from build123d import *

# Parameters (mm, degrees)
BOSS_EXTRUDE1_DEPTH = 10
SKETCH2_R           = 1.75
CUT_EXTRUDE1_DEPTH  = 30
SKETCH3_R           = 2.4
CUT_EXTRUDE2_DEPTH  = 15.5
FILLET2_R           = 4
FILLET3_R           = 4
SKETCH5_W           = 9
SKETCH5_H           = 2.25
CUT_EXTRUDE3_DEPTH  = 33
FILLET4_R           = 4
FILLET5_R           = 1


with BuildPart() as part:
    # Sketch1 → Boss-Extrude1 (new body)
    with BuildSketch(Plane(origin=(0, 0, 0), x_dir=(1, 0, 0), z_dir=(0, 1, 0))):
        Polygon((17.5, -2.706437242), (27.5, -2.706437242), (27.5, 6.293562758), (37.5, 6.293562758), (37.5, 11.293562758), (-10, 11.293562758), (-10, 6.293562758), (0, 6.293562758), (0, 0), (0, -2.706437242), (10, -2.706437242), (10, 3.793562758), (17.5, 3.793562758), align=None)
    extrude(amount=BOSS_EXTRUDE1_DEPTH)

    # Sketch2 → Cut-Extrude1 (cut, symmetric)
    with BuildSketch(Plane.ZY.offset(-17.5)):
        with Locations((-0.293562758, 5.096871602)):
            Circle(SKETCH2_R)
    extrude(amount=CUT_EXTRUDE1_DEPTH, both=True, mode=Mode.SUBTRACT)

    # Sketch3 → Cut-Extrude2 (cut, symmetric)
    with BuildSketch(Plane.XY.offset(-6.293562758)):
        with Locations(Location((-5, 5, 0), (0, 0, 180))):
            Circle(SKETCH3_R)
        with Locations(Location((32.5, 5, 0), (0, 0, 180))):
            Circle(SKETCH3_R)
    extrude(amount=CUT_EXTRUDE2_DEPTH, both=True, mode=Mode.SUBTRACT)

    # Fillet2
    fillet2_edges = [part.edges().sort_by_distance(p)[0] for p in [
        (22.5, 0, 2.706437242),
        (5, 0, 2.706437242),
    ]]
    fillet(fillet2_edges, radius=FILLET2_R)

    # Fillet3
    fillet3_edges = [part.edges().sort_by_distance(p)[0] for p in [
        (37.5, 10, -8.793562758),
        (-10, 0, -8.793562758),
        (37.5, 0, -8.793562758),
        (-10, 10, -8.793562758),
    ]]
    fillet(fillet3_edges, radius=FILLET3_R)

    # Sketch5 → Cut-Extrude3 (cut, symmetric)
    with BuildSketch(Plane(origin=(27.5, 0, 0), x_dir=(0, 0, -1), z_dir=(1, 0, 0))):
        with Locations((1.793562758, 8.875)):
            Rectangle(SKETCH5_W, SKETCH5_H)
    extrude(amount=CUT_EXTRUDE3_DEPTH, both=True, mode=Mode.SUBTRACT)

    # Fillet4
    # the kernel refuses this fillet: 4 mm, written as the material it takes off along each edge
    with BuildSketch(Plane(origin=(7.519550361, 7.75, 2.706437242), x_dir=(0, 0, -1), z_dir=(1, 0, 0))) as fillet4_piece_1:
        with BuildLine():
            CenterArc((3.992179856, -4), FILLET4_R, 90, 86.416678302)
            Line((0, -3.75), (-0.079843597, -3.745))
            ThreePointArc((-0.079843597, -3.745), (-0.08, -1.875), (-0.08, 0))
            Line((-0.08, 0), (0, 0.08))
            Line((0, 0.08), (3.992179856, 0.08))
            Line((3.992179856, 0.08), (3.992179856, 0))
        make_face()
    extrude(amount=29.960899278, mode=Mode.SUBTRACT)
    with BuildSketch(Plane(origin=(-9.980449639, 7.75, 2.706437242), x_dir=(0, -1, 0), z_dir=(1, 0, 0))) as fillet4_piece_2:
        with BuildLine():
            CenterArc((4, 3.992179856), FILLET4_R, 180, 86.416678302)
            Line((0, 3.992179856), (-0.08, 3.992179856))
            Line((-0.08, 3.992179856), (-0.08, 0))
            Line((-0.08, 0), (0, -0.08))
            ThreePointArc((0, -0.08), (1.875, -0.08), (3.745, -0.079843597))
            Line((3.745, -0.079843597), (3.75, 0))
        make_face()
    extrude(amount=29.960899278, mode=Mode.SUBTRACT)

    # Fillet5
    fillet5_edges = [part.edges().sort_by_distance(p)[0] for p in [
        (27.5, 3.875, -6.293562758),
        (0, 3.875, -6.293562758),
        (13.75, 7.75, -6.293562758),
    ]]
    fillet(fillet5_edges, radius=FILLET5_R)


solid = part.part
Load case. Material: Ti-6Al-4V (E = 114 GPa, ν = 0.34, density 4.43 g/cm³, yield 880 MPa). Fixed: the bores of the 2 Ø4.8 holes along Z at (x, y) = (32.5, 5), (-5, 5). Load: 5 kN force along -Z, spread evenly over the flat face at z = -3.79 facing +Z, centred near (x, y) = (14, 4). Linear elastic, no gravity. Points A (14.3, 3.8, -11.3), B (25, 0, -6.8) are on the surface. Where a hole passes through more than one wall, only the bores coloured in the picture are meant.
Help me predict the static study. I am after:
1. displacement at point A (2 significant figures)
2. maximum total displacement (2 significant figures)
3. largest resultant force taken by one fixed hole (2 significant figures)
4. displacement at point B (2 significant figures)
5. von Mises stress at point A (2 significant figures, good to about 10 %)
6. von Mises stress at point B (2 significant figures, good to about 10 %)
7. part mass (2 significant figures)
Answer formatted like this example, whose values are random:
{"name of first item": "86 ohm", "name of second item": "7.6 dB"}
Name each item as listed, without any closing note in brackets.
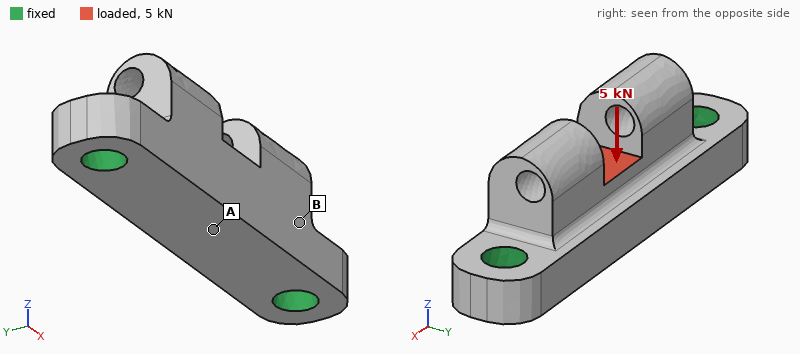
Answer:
{"displacement at point A": "56 µm", "maximum total displacement": "68 µm", "largest resultant force taken by one fixed hole": "3.1 kN", "displacement at point B": "26 µm", "von Mises stress at point A": "240 MPa", "von Mises stress at point B": "95 MPa", "part mass": "15 g"}
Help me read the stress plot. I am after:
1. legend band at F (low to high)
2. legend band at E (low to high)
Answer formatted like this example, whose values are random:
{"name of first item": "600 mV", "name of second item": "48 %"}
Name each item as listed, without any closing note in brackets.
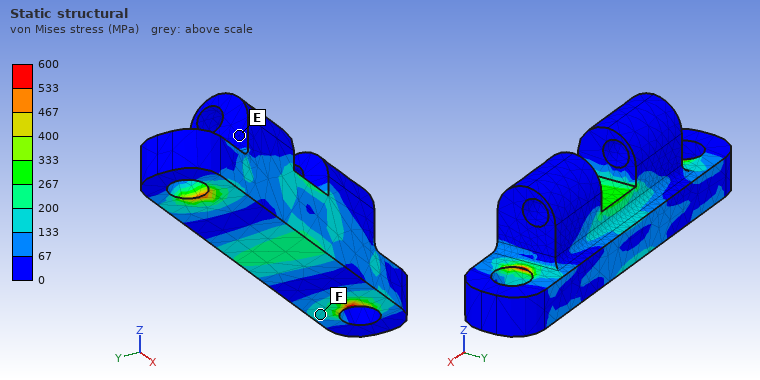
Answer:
{"legend band at F": "133 to 200 MPa", "legend band at E": "0 to 67 MPa"}
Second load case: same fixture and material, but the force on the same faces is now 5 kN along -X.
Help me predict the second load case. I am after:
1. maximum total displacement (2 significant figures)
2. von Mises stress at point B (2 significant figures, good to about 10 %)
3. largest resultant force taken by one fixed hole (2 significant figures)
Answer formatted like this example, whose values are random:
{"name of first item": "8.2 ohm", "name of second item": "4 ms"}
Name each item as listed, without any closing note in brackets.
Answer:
{"maximum total displacement": "11 µm", "von Mises stress at point B": "56 MPa", "largest resultant force taken by one fixed hole": "2.6 kN"}
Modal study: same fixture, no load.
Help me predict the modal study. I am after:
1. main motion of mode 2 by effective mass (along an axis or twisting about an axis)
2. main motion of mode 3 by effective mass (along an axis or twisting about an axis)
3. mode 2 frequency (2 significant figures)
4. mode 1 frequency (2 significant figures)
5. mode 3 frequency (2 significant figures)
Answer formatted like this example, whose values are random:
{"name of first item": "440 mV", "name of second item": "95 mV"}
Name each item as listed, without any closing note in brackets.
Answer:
{"main motion of mode 2 by effective mass": "along Z", "main motion of mode 3 by effective mass": "along Y", "mode 2 frequency": "19 kHz", "mode 1 frequency": "17 kHz", "mode 3 frequency": "27 kHz"}
